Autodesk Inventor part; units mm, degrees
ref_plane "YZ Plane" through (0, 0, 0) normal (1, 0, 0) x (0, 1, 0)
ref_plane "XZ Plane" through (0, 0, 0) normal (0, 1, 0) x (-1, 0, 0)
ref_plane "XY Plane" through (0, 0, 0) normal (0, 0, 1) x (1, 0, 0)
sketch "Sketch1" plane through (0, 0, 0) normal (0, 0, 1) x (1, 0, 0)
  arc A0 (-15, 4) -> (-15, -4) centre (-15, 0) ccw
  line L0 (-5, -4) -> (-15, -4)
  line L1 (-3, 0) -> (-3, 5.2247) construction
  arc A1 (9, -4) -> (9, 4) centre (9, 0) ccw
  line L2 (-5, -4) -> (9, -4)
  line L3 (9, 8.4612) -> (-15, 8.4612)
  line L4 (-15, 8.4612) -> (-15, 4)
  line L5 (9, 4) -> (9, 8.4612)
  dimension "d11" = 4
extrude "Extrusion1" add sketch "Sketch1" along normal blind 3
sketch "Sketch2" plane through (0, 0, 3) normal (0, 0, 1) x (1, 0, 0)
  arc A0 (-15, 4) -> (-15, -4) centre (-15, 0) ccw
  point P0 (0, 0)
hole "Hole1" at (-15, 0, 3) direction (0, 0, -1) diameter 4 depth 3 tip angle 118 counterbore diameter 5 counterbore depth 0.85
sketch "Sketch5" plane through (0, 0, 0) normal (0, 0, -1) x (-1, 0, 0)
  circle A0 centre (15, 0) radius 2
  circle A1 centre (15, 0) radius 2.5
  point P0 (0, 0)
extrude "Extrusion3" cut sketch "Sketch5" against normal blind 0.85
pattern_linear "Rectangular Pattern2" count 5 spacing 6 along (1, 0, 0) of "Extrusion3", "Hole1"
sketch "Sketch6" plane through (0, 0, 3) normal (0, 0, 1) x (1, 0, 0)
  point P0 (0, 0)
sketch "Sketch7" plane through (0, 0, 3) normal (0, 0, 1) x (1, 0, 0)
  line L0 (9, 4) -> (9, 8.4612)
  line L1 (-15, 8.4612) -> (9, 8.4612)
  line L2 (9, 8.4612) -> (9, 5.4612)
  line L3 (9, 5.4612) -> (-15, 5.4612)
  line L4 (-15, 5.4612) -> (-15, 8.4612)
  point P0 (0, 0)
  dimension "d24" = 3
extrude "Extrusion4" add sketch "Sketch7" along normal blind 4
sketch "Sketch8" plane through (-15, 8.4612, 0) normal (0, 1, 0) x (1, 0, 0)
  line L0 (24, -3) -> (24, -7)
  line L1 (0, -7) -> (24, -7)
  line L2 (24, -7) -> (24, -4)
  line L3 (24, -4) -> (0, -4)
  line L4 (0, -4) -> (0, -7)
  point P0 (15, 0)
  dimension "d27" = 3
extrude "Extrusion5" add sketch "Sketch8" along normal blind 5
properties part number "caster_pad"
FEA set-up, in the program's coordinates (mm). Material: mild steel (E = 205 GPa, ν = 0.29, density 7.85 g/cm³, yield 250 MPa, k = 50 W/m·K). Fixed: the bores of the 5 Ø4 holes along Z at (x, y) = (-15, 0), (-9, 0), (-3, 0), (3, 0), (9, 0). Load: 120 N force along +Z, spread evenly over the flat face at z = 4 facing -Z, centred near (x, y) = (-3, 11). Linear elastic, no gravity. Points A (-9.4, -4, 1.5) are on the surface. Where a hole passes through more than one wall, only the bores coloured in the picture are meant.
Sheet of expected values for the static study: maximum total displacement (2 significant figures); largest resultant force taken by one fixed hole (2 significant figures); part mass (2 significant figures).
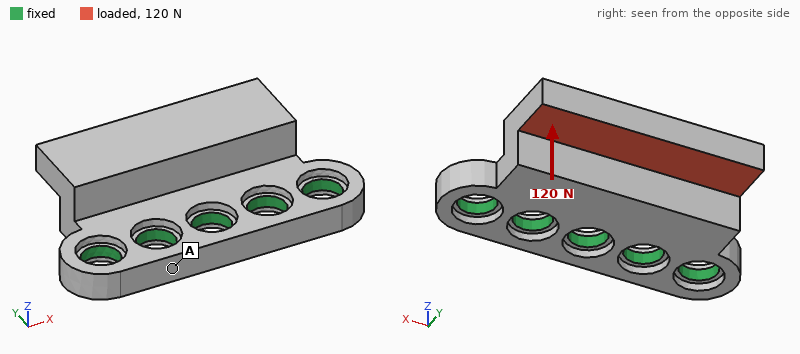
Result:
10 µm
30 N
11 g
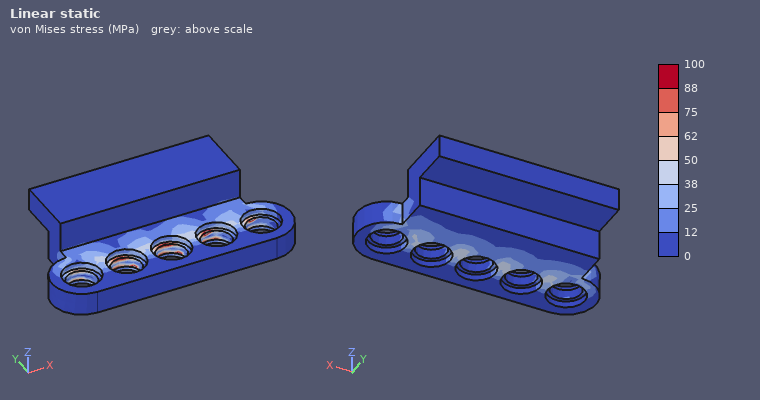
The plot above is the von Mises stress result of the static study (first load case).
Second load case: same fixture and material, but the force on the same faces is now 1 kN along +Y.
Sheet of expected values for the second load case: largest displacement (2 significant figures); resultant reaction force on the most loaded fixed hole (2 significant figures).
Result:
22 µm
260 N
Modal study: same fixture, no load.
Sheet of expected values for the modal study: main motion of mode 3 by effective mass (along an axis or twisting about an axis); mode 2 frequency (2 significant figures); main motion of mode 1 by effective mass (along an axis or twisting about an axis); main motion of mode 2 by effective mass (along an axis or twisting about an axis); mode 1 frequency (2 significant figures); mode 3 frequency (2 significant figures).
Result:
along X
20 kHz
along Z
twisting about Y
9500 Hz
40 kHz
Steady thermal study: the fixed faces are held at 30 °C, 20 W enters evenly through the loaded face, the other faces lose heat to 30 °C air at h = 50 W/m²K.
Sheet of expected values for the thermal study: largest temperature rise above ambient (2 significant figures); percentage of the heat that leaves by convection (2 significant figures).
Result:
63 K
7.3 %
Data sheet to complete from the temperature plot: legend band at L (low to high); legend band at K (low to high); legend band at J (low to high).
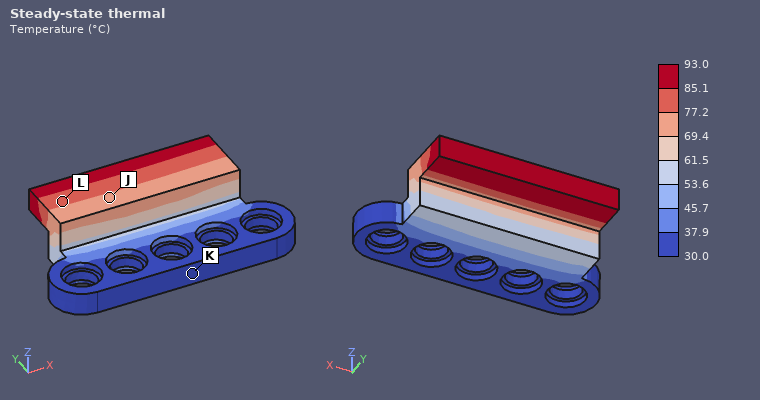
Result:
77.2 to 85.1 °C
30.0 to 37.9 °C
69.4 to 77.2 °C
